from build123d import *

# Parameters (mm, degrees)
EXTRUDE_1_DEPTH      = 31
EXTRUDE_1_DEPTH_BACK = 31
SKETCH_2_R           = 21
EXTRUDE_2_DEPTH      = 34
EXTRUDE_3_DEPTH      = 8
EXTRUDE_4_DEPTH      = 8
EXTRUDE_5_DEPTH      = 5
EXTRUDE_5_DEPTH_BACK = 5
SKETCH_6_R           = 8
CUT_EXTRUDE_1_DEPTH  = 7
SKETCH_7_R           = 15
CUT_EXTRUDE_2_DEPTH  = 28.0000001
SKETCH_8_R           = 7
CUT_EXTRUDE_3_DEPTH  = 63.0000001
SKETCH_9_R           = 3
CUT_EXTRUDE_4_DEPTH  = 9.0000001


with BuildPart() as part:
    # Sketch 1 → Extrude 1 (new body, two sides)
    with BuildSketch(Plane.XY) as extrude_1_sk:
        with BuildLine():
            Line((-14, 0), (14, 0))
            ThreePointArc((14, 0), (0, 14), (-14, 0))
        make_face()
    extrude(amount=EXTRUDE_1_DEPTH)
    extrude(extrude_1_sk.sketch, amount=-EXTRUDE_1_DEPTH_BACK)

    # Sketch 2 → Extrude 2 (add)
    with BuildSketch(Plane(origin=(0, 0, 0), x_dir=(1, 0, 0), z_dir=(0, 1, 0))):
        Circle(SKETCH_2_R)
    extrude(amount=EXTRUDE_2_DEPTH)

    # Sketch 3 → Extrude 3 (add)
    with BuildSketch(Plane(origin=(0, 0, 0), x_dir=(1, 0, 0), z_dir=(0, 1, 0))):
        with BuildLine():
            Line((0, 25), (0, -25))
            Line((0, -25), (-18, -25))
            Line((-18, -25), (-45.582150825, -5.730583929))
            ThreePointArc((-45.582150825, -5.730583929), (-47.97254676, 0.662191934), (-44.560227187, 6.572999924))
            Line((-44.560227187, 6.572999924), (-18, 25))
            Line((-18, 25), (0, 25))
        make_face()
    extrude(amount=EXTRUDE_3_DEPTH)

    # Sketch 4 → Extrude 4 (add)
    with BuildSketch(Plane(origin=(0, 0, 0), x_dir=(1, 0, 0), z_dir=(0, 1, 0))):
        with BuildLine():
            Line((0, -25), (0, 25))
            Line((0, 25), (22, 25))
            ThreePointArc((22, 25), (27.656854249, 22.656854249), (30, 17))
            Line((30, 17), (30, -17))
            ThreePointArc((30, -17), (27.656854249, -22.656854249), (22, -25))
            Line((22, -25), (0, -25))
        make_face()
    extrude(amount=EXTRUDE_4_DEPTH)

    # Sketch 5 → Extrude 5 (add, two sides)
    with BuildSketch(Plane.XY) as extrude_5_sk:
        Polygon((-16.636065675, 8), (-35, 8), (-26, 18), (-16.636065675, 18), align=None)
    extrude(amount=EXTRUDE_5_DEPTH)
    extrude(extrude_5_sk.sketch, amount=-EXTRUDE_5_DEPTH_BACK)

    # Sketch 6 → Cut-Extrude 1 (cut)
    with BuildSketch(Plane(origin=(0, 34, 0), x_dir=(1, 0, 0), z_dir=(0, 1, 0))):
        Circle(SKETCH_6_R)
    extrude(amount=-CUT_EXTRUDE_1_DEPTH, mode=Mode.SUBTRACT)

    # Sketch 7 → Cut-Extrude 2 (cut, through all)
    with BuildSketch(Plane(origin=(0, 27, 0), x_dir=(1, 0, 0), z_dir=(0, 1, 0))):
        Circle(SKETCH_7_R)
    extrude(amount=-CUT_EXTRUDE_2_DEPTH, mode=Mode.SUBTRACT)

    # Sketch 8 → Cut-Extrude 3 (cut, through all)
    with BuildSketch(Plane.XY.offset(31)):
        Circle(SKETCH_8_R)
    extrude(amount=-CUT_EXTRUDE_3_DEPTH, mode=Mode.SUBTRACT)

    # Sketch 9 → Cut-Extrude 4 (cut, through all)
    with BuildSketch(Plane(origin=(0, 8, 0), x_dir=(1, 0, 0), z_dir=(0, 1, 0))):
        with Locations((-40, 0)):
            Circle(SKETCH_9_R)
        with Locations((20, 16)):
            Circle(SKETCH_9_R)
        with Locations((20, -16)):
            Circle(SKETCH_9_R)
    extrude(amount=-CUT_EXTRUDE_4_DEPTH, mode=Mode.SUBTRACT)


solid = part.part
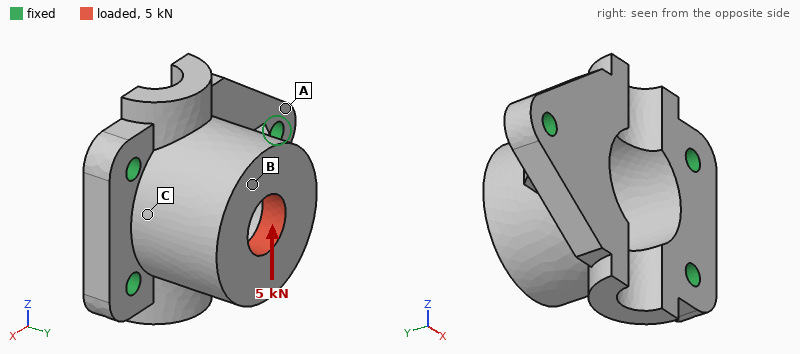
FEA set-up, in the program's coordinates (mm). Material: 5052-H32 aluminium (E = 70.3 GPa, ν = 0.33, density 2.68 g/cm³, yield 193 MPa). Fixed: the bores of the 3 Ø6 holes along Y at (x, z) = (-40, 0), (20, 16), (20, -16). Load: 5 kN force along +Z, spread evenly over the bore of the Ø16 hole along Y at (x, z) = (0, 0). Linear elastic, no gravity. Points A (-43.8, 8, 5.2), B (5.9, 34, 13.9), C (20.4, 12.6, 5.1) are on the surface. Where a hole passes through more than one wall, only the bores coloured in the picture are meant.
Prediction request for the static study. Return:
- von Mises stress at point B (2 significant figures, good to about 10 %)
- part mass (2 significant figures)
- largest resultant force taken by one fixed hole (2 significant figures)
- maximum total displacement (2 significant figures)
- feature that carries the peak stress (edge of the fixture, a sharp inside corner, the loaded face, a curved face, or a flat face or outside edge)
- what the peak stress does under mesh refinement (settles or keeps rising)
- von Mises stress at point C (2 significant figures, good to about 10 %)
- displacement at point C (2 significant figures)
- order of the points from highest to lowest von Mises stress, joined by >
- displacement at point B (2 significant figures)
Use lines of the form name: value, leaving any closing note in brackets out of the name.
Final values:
von Mises stress at point B: 21 MPa
part mass: 120 g
largest resultant force taken by one fixed hole: 4.4 kN
maximum total displacement: 57 µm
feature that carries the peak stress: edge of the fixture
what the peak stress does under mesh refinement: keeps rising
von Mises stress at point C: 40 MPa
displacement at point C: 12 µm
order of the points from highest to lowest von Mises stress, joined by >: C > B > A
displacement at point B: 52 µm
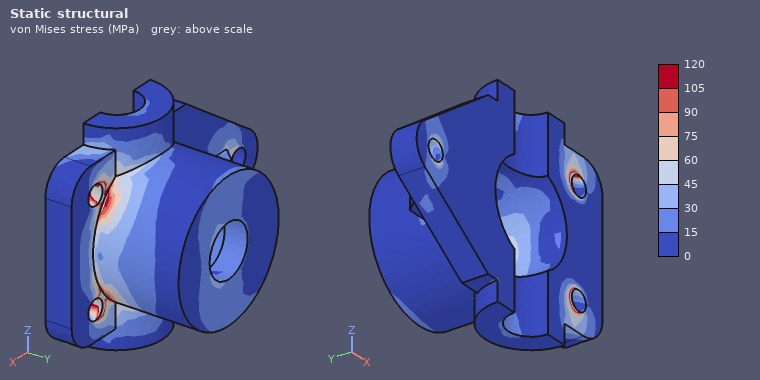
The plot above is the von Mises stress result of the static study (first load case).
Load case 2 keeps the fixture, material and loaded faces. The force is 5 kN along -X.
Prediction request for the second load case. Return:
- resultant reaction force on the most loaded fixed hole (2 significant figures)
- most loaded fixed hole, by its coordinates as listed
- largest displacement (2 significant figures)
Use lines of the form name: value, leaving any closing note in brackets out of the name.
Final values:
resultant reaction force on the most loaded fixed hole: 3.5 kN
most loaded fixed hole, by its coordinates as listed: (-40, 0)
largest displacement: 35 µm
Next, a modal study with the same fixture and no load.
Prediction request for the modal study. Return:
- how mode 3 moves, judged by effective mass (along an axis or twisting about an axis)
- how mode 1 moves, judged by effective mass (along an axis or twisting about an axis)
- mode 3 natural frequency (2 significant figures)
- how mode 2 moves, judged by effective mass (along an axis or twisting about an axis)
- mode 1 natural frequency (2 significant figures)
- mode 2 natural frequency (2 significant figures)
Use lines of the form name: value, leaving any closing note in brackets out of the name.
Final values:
how mode 3 moves, judged by effective mass: along Z
how mode 1 moves, judged by effective mass: along Z
mode 3 natural frequency: 12 kHz
how mode 2 moves, judged by effective mass: along Y
mode 1 natural frequency: 7500 Hz
mode 2 natural frequency: 8600 Hz
